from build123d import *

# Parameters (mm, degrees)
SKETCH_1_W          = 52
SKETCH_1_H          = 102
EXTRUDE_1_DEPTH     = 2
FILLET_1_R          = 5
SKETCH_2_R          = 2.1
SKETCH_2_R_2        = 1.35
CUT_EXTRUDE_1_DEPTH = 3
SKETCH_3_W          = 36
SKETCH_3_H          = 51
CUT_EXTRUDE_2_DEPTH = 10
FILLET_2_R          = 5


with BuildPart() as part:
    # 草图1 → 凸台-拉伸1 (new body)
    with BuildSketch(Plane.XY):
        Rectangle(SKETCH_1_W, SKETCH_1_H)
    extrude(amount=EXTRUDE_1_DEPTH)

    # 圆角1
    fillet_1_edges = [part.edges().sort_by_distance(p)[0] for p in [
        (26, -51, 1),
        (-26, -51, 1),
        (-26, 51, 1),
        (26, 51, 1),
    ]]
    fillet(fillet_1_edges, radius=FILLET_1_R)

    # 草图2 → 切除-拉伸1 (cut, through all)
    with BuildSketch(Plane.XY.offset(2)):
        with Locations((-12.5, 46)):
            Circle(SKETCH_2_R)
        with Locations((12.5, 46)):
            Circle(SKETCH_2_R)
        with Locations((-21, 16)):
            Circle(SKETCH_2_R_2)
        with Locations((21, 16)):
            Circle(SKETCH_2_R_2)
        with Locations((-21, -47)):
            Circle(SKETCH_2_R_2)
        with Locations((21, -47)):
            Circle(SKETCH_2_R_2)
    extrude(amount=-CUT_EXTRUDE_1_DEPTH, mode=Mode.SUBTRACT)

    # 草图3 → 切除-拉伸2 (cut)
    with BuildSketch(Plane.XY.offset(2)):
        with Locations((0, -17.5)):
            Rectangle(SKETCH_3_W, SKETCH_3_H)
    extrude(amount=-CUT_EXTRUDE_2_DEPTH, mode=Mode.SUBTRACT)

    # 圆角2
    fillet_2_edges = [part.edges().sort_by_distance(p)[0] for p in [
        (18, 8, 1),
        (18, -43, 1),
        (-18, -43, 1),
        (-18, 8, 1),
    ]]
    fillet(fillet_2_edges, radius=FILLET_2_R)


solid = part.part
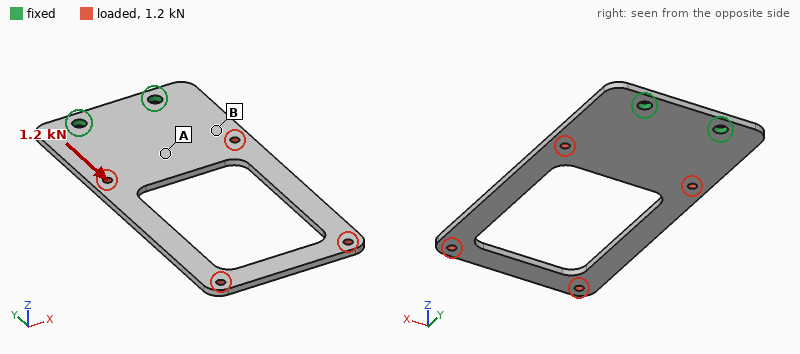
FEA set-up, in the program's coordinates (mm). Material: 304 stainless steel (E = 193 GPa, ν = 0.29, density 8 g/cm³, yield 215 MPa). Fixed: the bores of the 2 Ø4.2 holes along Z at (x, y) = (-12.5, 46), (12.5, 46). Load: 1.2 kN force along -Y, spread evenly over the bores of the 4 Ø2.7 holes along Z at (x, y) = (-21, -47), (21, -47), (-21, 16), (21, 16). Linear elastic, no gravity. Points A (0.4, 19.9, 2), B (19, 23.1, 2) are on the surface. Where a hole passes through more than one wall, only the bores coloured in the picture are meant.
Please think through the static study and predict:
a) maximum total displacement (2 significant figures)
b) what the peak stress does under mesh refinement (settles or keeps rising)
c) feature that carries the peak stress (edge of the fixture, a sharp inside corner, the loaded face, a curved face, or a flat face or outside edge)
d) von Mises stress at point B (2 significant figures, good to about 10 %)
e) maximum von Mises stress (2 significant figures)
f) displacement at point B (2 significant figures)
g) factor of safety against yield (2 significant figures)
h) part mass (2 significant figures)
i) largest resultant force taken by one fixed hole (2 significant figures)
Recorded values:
12 µm
settles
the loaded face
20 MPa
68 MPa
2.4 µm
3.1
55 g
600 N
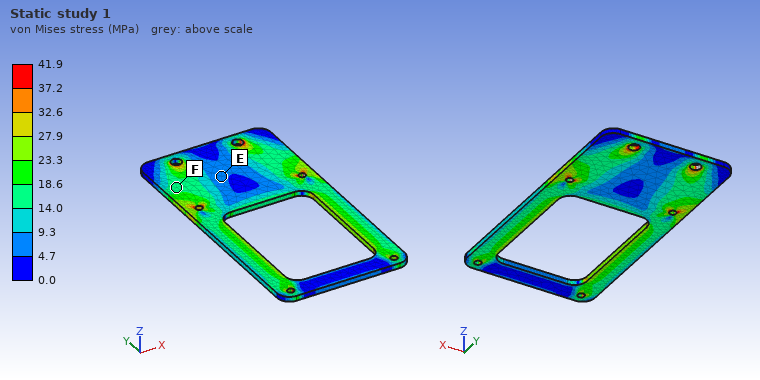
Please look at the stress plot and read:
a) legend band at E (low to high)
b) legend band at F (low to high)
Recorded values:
4.7 to 9.3 MPa
14.0 to 18.6 MPa
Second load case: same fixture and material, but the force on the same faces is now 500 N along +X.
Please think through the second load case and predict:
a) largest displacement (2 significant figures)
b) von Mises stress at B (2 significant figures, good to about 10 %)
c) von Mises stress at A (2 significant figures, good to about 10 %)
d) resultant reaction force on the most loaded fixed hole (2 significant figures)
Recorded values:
0.18 mm
13 MPa
25 MPa
1.1 kN
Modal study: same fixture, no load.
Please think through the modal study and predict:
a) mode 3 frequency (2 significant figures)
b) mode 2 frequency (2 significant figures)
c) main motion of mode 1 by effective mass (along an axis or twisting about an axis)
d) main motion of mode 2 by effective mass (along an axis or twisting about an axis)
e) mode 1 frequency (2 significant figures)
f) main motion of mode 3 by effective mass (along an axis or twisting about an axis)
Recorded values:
990 Hz
580 Hz
along Z
twisting about Y
200 Hz
along Z
